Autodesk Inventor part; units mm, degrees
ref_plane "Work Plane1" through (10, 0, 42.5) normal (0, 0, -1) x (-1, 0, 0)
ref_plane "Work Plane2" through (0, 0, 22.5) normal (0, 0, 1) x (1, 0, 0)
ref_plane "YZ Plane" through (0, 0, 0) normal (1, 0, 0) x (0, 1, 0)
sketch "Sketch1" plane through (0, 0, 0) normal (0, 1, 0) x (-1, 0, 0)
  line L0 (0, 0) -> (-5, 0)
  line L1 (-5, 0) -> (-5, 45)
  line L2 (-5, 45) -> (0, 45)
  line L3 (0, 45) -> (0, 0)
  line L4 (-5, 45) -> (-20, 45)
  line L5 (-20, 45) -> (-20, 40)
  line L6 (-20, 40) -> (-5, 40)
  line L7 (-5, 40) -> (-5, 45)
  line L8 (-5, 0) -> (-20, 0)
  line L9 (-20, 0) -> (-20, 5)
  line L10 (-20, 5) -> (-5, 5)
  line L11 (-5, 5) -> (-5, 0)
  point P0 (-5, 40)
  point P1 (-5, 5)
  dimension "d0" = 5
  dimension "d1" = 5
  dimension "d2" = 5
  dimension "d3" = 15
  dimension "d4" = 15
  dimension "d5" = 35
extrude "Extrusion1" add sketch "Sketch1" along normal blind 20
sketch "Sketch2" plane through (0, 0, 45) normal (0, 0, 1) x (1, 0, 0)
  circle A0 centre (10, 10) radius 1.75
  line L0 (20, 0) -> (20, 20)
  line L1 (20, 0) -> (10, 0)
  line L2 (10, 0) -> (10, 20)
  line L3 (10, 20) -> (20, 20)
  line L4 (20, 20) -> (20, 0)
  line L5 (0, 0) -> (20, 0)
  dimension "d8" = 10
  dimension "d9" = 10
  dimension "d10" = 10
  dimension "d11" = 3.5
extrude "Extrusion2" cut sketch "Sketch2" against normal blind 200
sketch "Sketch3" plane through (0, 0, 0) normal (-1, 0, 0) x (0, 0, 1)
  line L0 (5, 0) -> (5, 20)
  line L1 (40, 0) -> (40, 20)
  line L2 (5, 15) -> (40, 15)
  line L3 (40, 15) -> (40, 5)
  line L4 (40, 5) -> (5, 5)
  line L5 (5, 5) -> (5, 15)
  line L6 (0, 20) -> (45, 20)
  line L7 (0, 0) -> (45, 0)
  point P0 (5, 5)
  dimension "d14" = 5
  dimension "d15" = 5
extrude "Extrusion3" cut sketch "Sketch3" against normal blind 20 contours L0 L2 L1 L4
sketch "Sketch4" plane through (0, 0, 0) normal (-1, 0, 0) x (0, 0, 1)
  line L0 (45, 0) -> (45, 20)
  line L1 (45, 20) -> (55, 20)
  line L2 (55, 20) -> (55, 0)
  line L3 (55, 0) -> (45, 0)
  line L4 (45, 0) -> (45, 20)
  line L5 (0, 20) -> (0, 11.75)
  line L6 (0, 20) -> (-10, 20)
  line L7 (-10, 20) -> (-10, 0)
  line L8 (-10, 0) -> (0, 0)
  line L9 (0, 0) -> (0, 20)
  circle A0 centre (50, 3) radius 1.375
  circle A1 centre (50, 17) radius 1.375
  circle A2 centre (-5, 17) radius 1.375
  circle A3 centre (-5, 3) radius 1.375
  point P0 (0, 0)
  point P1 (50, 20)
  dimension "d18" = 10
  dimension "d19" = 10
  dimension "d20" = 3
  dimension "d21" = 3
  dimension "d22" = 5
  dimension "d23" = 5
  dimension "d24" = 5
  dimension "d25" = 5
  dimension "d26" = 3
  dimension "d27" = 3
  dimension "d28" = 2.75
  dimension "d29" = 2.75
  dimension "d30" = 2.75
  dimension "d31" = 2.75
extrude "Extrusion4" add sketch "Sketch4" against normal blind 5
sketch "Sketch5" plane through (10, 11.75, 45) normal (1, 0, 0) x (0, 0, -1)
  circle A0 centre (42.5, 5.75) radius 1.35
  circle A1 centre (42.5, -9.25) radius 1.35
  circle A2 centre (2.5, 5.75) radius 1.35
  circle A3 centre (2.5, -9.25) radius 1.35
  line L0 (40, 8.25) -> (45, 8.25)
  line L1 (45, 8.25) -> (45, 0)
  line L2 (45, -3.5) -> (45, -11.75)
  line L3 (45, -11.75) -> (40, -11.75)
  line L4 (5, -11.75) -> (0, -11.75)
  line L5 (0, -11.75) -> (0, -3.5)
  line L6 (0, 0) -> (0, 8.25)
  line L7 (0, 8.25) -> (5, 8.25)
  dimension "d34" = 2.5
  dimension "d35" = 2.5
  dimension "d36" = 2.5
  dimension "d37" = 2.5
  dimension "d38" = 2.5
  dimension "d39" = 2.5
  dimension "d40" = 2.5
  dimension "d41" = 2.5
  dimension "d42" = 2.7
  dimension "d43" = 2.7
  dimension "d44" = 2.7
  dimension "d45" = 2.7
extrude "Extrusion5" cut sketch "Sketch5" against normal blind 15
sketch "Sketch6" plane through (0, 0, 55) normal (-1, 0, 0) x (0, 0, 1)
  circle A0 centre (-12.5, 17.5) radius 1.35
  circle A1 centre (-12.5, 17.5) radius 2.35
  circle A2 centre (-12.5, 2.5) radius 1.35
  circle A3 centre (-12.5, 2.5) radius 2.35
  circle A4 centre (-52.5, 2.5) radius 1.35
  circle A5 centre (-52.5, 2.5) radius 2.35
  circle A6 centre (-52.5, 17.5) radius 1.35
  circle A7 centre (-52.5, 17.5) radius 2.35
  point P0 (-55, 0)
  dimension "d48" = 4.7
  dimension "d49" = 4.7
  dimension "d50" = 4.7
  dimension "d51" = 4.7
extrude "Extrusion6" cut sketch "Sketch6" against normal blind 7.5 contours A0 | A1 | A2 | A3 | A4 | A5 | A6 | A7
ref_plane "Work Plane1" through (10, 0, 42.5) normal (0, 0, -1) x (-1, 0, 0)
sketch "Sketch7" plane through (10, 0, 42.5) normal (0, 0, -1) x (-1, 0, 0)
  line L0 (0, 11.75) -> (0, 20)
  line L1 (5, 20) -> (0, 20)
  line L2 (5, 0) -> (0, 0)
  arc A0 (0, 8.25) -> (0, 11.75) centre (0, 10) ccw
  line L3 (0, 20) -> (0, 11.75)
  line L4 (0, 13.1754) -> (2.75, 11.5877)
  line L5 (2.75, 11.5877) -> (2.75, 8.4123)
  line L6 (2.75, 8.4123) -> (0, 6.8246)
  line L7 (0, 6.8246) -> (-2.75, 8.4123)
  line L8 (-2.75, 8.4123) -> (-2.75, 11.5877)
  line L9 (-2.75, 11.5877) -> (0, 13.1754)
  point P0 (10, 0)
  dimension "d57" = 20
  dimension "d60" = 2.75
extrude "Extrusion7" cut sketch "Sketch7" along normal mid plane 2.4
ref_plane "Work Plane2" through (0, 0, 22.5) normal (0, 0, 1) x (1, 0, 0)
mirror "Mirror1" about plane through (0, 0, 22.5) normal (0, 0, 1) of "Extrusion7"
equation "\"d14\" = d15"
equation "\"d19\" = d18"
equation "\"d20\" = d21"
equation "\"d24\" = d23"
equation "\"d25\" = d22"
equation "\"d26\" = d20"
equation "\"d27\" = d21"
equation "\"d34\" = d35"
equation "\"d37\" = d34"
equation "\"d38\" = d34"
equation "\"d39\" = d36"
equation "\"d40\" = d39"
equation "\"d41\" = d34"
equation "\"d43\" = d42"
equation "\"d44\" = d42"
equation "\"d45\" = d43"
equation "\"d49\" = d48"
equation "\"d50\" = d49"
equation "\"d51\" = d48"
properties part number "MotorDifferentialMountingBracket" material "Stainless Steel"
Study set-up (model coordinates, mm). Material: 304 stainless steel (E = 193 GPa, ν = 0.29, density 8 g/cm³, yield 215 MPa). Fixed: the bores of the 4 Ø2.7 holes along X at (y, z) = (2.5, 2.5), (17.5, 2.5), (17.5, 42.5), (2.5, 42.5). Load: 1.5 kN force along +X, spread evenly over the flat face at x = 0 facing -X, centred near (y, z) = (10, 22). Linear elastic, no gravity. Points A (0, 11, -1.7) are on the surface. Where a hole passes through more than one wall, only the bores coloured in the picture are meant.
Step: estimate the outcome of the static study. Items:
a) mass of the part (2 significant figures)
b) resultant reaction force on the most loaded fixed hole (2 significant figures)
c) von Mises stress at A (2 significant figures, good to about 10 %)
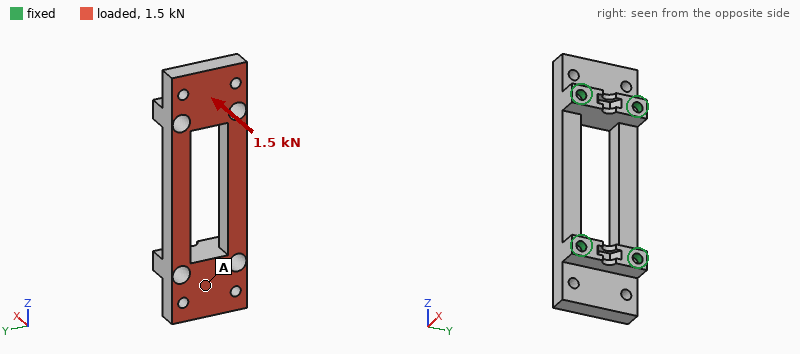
40 g
390 N
18 MPa
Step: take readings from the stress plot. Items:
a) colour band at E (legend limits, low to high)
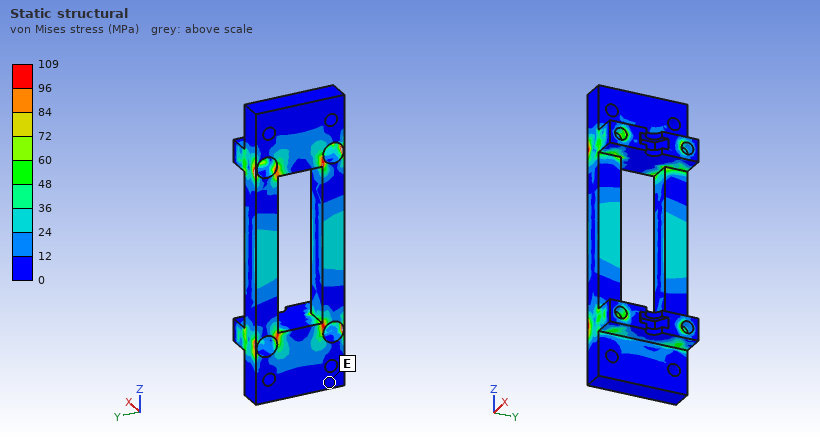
0 to 12 MPa
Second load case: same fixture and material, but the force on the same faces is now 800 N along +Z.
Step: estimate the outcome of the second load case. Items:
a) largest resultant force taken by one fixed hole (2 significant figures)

200 N
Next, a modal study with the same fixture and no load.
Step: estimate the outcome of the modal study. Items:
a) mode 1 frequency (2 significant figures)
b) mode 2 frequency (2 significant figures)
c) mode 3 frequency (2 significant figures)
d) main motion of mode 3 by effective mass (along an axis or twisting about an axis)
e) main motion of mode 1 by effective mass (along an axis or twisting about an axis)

9300 Hz
10 kHz
12 kHz
twisting about Z
along Z
